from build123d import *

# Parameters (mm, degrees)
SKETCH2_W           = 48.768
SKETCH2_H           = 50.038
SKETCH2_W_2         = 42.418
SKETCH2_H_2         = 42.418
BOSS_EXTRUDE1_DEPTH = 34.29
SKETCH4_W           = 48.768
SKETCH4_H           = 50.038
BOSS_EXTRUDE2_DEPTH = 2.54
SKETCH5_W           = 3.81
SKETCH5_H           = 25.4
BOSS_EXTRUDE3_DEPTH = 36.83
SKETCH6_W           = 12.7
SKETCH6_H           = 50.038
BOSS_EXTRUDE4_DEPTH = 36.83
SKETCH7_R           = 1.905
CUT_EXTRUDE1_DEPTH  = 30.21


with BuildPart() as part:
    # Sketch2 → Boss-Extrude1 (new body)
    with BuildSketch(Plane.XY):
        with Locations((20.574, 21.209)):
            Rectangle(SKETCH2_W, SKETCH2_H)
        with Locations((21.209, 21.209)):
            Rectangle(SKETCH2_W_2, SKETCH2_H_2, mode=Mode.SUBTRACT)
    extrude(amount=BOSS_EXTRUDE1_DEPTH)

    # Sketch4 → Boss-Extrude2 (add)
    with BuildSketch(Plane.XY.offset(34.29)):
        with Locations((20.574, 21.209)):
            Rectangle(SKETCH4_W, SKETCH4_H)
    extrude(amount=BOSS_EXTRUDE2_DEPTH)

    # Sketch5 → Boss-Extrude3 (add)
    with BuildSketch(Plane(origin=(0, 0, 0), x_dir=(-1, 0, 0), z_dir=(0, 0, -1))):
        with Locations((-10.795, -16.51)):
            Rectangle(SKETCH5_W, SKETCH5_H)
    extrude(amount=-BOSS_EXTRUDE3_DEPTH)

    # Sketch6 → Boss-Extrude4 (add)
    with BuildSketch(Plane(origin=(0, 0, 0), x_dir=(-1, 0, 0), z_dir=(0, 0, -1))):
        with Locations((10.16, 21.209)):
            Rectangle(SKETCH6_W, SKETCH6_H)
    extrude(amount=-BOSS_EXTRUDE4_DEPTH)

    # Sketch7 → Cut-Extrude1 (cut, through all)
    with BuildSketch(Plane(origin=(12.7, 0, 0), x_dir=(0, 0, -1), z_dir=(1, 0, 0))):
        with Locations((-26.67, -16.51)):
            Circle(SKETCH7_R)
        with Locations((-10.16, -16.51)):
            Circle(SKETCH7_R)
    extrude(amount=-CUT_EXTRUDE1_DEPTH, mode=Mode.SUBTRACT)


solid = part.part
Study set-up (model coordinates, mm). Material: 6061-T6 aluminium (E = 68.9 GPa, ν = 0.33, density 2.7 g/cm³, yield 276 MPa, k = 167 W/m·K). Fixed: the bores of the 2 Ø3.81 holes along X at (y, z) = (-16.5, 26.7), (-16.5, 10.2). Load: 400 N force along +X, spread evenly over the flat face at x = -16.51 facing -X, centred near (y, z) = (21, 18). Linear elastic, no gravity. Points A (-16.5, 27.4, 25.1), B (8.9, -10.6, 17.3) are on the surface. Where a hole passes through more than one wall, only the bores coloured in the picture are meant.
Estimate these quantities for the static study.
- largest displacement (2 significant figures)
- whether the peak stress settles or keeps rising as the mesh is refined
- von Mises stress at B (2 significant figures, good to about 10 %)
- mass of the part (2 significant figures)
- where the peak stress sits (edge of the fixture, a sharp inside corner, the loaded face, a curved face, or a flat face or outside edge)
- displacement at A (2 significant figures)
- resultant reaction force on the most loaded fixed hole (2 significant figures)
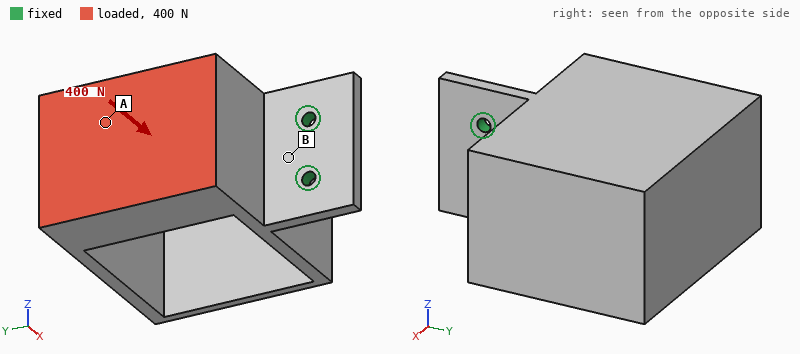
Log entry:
1.0 mm
keeps rising
120 MPa
150 g
edge of the fixture
0.73 mm
200 N
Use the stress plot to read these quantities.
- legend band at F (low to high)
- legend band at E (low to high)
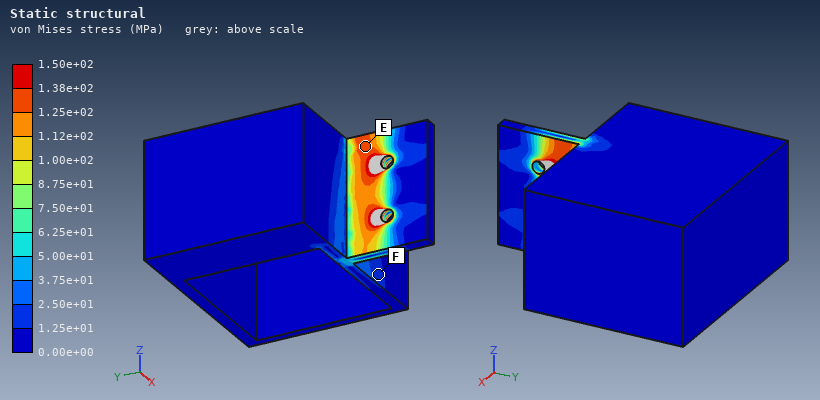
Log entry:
1.25e+01 to 2.50e+01 MPa
1.25e+02 to 1.38e+02 MPa
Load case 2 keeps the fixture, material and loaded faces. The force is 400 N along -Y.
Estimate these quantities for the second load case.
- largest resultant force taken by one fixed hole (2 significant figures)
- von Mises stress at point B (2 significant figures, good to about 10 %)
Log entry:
200 N
110 MPa
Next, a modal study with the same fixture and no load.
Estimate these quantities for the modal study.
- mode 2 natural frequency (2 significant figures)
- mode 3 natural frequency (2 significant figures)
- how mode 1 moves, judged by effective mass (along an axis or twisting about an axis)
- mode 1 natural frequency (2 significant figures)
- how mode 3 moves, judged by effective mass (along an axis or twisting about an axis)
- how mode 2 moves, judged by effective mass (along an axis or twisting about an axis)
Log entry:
1200 Hz
1300 Hz
along X
290 Hz
along Z
twisting about Y
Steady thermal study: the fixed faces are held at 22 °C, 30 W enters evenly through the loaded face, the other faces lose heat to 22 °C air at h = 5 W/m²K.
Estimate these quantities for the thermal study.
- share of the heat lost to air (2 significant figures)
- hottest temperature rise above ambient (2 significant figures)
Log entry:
8.1 %
34 K
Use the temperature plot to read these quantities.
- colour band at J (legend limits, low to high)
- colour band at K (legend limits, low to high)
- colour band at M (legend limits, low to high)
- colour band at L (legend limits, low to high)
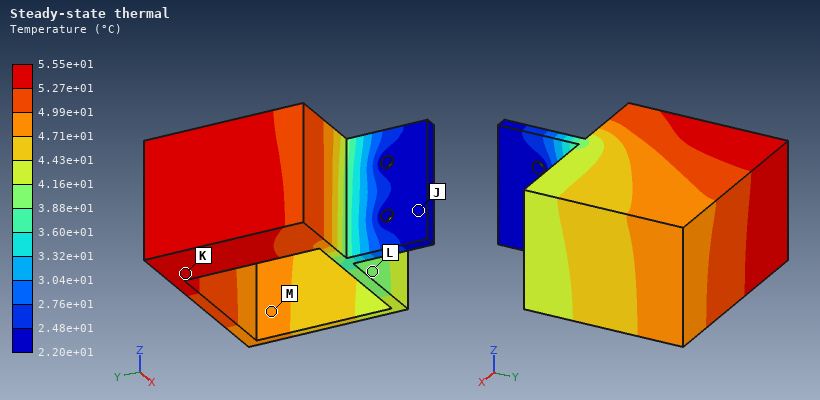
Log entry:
2.20e+01 to 2.48e+01 °C
5.27e+01 to 5.55e+01 °C
4.71e+01 to 4.99e+01 °C
3.88e+01 to 4.16e+01 °C
